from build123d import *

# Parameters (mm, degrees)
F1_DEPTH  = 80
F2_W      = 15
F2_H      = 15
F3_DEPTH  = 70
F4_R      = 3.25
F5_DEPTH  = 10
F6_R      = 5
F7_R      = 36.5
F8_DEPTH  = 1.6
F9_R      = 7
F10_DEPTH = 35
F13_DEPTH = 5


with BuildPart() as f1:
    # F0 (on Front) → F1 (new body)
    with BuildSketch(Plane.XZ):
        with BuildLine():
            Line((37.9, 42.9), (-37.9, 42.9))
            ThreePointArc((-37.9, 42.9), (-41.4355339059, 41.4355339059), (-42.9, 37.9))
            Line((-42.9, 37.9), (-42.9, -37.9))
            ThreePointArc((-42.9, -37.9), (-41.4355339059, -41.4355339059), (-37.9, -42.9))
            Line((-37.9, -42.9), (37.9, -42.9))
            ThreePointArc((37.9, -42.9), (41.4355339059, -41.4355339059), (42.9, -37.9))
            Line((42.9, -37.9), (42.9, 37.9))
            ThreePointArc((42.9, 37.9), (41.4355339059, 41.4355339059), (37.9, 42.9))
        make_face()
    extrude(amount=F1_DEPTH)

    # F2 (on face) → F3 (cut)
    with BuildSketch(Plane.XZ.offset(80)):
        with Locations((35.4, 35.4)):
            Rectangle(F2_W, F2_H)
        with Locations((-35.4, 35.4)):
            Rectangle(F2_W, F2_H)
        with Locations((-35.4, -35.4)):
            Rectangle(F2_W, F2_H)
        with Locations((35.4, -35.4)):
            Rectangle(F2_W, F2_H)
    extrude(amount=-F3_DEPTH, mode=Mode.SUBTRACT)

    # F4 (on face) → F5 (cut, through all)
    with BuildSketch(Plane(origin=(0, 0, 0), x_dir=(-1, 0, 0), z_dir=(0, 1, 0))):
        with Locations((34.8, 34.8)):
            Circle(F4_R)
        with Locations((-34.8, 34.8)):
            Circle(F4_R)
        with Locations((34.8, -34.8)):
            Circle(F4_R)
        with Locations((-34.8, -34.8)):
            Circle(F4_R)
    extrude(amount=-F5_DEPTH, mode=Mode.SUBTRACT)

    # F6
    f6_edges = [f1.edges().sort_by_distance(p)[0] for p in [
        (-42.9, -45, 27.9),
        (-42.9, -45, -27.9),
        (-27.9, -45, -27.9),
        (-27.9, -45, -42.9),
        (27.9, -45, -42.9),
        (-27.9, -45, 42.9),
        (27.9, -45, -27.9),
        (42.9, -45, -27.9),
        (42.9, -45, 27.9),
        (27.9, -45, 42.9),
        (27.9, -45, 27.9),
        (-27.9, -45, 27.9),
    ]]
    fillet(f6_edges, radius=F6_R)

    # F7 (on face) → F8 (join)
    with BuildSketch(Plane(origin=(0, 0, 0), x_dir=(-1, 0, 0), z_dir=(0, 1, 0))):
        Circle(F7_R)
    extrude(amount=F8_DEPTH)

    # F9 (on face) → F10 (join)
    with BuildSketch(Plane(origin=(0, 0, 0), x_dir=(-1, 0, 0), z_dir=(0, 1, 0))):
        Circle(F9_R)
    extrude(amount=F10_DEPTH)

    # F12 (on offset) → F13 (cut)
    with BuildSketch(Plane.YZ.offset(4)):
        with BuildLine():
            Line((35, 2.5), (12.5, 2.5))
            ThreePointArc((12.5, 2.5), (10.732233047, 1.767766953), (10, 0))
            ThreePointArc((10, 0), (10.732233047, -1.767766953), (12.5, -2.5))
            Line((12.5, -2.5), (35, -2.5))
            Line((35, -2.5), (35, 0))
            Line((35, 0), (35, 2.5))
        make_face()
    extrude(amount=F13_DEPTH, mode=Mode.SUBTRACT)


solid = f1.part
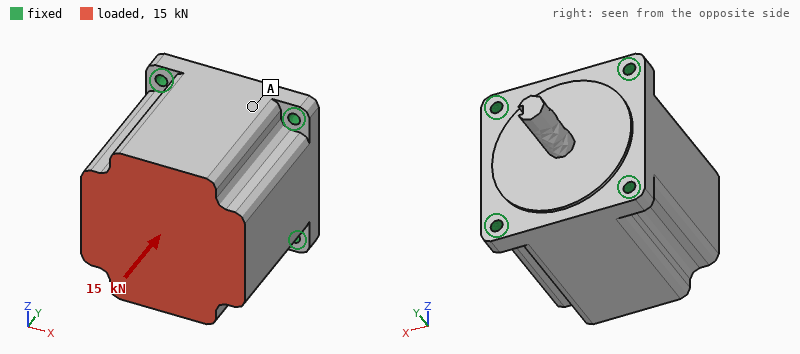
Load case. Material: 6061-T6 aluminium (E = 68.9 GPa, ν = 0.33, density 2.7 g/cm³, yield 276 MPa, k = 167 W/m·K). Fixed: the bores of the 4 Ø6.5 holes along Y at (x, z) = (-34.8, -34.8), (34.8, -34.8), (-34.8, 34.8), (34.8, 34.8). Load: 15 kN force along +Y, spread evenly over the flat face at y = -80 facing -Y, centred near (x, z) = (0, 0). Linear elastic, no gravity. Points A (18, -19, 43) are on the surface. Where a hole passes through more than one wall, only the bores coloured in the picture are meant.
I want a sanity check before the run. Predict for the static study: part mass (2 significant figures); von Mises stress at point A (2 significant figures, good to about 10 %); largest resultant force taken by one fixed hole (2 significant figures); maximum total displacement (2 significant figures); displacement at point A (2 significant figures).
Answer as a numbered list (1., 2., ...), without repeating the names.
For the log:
1. 1.4 kg
2. 6.8 MPa
3. 4.0 kN
4. 11 µm
5. 8.2 µm
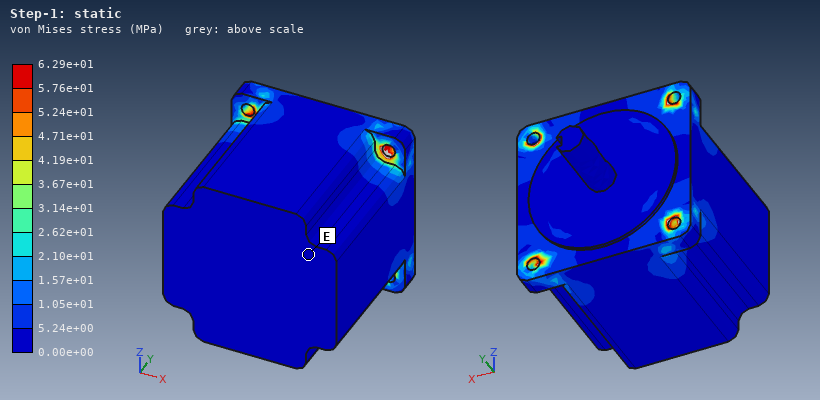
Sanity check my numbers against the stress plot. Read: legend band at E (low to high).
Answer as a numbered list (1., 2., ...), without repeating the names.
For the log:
1. 0.00e+00 to 5.24e+00 MPa
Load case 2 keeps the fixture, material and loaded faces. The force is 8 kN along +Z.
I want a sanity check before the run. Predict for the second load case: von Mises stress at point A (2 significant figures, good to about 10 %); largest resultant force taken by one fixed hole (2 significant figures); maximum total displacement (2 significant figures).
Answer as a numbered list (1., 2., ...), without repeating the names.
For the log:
1. 8.9 MPa
2. 5.1 kN
3. 35 µm
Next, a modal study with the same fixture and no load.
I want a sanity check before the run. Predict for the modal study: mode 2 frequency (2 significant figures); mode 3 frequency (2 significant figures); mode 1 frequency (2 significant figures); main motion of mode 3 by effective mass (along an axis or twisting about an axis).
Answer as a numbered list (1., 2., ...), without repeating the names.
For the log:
1. 3500 Hz
2. 5400 Hz
3. 3500 Hz
4. along Y
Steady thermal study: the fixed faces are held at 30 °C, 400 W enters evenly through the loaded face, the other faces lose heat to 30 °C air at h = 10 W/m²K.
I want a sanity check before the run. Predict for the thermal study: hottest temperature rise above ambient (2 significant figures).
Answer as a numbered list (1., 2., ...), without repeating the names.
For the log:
1. 52 K
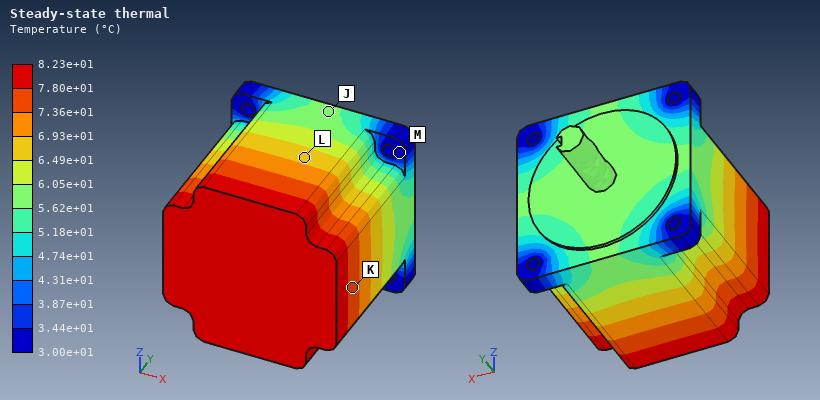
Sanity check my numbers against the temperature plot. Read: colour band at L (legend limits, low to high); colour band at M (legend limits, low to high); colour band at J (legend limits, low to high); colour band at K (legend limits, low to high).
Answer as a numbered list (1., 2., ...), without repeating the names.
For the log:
1. 6.49e+01 to 6.93e+01 °C
2. 3.00e+01 to 3.44e+01 °C
3. 5.62e+01 to 6.05e+01 °C
4. 7.36e+01 to 7.80e+01 °C
